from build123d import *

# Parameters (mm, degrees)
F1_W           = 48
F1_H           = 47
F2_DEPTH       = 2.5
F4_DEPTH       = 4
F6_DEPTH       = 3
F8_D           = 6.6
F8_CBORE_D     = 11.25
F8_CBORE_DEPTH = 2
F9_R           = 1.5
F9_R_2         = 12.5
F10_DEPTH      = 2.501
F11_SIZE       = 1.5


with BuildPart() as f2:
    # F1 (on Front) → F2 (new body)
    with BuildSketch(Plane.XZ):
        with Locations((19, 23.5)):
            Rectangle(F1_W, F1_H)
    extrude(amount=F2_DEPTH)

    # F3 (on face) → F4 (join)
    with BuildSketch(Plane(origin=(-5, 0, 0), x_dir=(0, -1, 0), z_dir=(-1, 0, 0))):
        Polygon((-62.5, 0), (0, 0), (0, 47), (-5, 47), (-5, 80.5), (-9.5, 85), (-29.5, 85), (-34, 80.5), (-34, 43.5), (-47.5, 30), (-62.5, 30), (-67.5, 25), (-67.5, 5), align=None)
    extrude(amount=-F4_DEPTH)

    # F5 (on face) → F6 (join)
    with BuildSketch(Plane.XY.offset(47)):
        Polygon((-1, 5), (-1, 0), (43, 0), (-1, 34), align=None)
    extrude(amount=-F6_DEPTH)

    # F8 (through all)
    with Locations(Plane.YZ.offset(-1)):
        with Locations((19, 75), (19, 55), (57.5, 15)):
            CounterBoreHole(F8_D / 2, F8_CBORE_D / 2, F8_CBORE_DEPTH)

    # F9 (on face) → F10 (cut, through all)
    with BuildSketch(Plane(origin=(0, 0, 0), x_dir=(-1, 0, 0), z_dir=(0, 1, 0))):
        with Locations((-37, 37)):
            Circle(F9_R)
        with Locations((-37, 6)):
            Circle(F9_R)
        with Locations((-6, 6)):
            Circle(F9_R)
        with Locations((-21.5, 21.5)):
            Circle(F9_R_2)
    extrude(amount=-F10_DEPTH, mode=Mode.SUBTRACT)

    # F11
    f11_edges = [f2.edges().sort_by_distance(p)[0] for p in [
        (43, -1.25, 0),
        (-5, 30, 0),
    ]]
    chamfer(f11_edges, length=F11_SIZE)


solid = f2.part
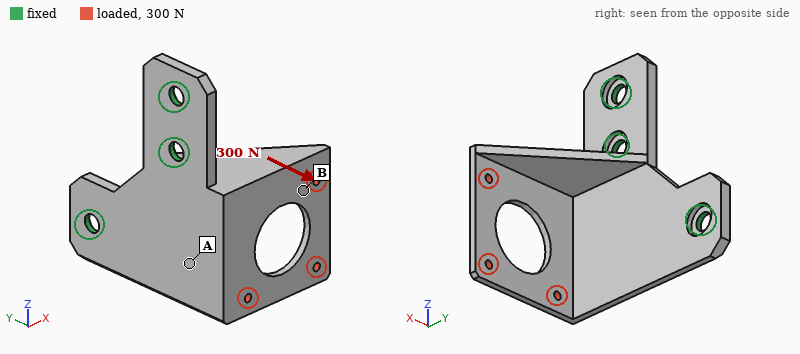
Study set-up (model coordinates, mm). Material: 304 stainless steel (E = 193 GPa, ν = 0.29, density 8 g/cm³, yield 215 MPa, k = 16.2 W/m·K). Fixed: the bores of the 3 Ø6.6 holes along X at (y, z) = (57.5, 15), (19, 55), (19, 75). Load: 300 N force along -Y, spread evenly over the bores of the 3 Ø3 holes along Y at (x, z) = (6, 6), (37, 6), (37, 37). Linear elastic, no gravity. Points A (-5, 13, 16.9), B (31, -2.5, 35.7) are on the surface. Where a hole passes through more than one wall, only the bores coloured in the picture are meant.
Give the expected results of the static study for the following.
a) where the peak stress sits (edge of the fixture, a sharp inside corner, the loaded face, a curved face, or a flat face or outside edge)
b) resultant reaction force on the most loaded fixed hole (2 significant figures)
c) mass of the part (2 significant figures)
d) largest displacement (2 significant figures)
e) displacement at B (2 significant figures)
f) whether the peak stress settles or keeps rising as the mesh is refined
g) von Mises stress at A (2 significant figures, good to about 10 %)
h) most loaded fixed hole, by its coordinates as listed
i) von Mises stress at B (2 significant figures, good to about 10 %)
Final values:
edge of the fixture
380 N
170 g
0.41 mm
0.11 mm
keeps rising
18 MPa
(57.5, 15)
78 MPa
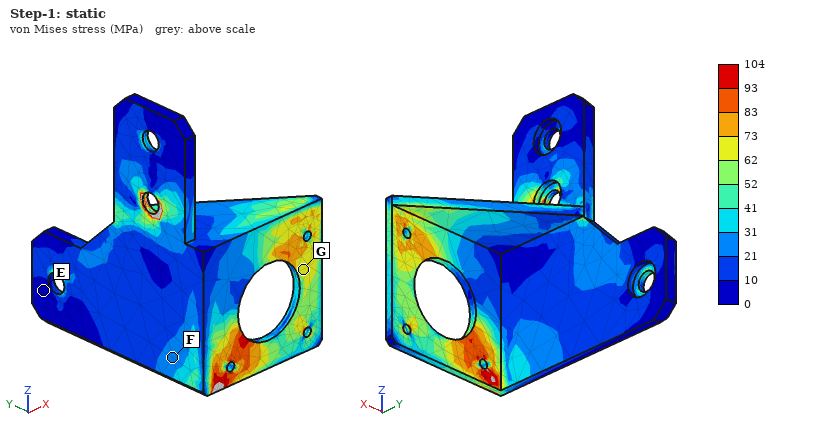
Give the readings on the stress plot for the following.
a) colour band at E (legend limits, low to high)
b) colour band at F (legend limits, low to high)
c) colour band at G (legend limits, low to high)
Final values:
0 to 10 MPa
21 to 31 MPa
62 to 73 MPa
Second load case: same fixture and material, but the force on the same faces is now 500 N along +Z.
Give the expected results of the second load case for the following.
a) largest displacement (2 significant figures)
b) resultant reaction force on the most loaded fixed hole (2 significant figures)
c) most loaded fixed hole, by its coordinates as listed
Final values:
0.37 mm
560 N
(19, 75)
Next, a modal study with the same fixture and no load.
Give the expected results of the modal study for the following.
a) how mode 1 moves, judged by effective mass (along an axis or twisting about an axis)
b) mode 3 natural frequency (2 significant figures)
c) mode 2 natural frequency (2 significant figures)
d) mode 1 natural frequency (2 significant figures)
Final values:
along X
2500 Hz
1400 Hz
850 Hz
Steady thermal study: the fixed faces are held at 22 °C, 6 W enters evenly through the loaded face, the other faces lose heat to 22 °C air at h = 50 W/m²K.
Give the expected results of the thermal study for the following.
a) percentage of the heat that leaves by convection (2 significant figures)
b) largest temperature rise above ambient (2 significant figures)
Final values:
94 %
55 K
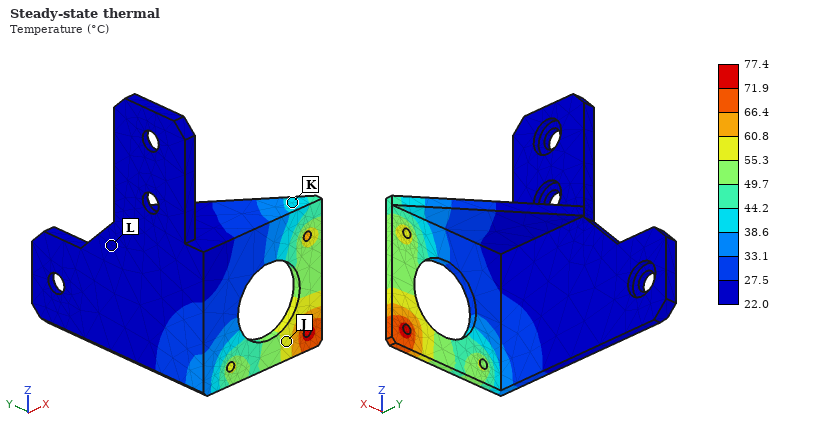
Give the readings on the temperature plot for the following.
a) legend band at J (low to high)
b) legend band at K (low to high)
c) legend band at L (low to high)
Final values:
55.3 to 60.8 °C
38.6 to 44.2 °C
22.0 to 27.5 °C
